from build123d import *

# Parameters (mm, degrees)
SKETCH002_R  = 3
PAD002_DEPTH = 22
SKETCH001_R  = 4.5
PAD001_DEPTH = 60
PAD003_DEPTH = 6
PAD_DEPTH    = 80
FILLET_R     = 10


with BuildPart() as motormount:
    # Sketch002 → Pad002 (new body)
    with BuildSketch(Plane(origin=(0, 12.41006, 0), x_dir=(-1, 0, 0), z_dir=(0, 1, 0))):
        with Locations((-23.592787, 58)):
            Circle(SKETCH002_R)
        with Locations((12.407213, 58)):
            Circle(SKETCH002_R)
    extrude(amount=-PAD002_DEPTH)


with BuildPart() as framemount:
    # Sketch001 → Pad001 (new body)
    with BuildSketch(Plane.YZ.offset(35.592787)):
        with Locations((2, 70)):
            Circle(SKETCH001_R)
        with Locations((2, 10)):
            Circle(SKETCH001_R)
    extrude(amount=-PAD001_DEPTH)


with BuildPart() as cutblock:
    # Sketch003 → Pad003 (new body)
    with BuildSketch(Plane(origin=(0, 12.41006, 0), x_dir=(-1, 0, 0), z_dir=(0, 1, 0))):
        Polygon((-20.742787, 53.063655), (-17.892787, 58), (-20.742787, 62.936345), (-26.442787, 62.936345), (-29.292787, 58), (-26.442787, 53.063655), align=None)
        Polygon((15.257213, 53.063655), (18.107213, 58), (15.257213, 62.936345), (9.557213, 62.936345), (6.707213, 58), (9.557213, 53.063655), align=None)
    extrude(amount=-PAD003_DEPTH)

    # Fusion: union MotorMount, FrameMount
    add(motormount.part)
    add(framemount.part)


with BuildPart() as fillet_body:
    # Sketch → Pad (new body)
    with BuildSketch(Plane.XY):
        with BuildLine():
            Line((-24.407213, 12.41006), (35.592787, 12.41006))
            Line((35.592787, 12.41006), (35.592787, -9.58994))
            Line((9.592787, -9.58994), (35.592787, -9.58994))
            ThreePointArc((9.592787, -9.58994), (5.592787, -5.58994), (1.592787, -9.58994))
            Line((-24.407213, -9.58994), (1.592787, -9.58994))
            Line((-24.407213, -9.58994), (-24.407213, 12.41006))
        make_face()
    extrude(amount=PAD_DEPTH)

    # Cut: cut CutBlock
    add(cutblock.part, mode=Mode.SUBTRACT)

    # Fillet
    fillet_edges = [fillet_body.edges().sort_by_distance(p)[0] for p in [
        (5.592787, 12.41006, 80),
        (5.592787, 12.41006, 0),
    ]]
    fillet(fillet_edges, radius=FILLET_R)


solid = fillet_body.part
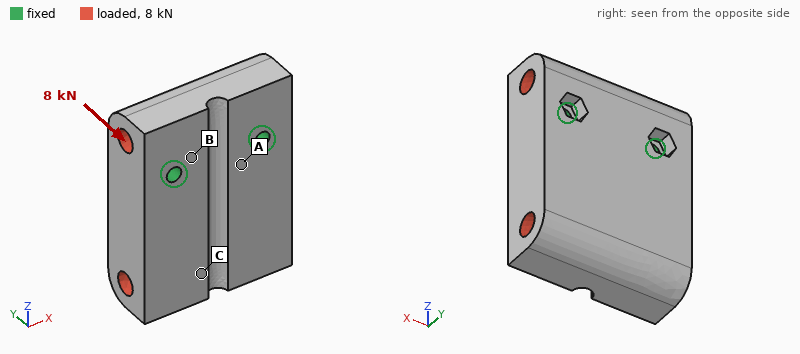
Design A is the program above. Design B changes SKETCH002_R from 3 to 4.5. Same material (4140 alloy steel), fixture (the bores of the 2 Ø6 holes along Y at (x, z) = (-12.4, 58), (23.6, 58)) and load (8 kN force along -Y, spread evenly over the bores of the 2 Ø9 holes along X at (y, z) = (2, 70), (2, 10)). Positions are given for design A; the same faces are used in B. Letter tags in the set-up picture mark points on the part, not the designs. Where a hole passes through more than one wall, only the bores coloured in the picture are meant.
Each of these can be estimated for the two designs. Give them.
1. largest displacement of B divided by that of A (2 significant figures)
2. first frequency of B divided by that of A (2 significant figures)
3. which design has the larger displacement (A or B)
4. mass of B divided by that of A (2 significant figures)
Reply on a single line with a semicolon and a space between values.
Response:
0.81; 1.2; A; 0.99
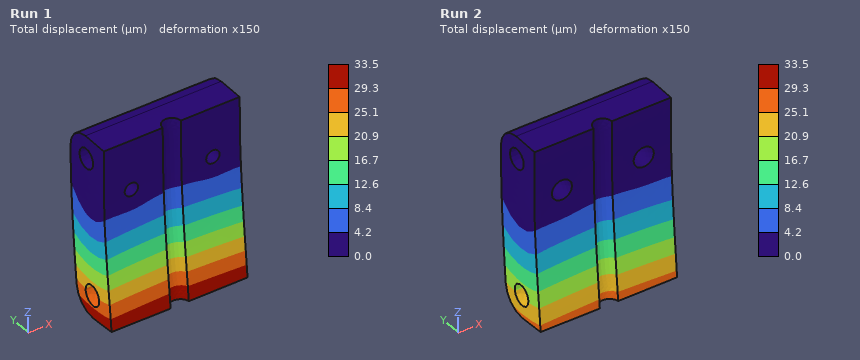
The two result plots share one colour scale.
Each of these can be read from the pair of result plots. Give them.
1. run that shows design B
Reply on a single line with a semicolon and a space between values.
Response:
Run 2
